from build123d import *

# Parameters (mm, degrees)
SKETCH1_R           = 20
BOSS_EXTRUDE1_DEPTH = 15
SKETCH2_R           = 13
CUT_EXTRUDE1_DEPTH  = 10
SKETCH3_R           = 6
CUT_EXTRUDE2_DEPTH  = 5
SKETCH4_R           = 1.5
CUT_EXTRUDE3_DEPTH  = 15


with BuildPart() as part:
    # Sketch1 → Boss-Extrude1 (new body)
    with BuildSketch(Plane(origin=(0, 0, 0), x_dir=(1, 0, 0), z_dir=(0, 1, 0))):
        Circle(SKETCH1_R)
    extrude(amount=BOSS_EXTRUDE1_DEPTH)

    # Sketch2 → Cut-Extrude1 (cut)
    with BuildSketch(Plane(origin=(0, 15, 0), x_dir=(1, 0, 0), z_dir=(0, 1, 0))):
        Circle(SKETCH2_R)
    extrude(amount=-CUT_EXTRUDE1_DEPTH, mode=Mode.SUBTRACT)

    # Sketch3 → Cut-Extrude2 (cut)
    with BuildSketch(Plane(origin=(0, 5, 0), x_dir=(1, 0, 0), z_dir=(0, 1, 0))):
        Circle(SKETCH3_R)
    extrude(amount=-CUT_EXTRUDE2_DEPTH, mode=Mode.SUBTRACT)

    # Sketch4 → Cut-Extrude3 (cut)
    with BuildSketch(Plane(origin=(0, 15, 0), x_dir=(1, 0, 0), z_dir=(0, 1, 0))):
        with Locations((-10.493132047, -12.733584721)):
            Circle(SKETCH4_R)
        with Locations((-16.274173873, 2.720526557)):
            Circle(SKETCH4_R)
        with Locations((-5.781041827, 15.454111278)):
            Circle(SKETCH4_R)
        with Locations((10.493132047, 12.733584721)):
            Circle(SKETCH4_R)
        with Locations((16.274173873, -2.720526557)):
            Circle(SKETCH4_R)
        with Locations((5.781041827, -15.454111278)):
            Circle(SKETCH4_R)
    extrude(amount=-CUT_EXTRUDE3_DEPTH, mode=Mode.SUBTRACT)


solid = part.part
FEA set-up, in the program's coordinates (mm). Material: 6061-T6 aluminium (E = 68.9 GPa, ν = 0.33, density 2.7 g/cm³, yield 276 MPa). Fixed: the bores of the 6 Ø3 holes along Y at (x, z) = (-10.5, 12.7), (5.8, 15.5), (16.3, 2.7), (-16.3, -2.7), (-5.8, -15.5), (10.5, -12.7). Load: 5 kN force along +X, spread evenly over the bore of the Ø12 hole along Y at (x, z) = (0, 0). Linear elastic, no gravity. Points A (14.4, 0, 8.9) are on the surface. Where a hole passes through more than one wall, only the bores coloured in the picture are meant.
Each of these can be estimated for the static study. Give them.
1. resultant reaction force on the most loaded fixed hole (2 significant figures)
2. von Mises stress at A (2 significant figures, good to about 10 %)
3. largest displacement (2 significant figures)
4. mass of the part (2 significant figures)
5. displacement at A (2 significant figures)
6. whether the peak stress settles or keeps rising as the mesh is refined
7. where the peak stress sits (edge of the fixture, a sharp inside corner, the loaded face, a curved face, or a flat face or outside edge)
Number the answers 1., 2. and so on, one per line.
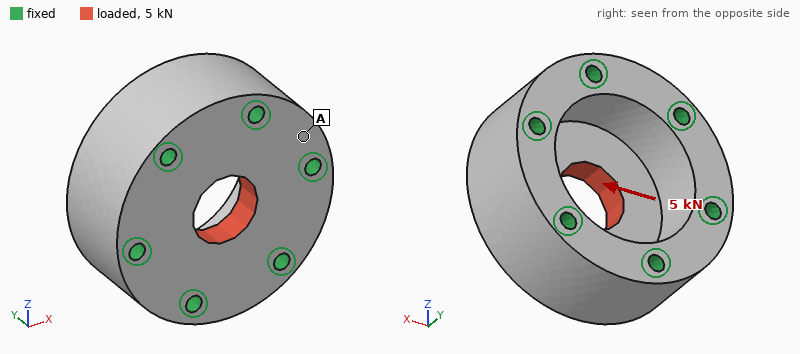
1. 1.2 kN
2. 5.9 MPa
3. 4.5 µm
4. 33 g
5. 1.7 µm
6. keeps rising
7. edge of the fixture
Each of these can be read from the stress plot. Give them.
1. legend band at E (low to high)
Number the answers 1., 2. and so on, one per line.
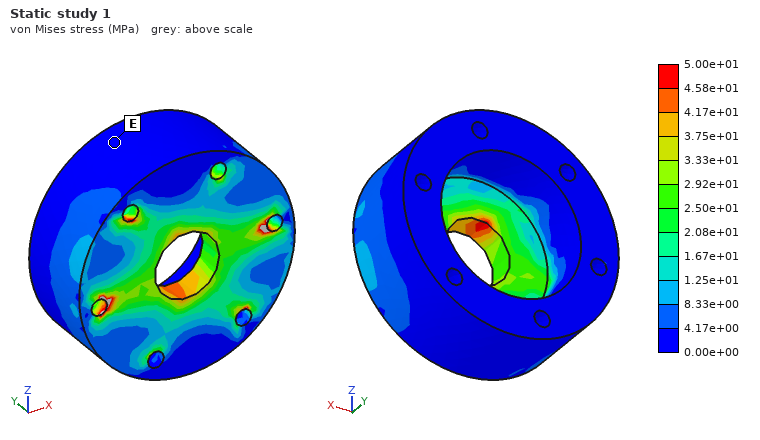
1. 0.00e+00 to 4.17e+00 MPa
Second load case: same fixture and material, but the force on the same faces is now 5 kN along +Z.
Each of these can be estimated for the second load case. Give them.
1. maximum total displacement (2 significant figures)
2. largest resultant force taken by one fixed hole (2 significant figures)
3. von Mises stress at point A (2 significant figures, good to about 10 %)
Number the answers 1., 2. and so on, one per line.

1. 4.5 µm
2. 1.2 kN
3. 5.7 MPa
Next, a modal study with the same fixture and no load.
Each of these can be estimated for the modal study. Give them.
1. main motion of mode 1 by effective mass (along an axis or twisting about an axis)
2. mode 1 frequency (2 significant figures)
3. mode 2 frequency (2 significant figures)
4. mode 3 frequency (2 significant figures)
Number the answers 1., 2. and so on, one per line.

1. along Y
2. 53 kHz
3. 66 kHz
4. 66 kHz
